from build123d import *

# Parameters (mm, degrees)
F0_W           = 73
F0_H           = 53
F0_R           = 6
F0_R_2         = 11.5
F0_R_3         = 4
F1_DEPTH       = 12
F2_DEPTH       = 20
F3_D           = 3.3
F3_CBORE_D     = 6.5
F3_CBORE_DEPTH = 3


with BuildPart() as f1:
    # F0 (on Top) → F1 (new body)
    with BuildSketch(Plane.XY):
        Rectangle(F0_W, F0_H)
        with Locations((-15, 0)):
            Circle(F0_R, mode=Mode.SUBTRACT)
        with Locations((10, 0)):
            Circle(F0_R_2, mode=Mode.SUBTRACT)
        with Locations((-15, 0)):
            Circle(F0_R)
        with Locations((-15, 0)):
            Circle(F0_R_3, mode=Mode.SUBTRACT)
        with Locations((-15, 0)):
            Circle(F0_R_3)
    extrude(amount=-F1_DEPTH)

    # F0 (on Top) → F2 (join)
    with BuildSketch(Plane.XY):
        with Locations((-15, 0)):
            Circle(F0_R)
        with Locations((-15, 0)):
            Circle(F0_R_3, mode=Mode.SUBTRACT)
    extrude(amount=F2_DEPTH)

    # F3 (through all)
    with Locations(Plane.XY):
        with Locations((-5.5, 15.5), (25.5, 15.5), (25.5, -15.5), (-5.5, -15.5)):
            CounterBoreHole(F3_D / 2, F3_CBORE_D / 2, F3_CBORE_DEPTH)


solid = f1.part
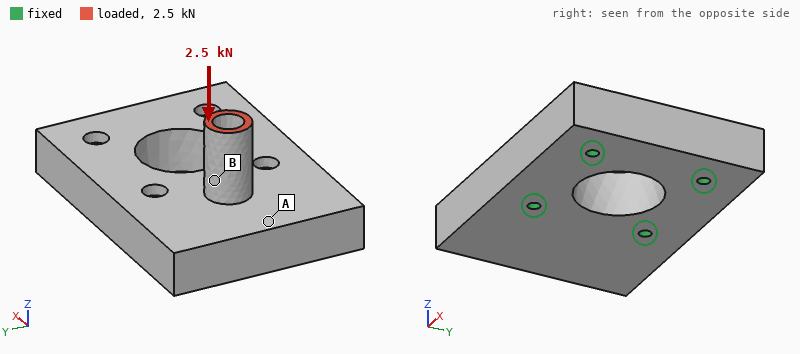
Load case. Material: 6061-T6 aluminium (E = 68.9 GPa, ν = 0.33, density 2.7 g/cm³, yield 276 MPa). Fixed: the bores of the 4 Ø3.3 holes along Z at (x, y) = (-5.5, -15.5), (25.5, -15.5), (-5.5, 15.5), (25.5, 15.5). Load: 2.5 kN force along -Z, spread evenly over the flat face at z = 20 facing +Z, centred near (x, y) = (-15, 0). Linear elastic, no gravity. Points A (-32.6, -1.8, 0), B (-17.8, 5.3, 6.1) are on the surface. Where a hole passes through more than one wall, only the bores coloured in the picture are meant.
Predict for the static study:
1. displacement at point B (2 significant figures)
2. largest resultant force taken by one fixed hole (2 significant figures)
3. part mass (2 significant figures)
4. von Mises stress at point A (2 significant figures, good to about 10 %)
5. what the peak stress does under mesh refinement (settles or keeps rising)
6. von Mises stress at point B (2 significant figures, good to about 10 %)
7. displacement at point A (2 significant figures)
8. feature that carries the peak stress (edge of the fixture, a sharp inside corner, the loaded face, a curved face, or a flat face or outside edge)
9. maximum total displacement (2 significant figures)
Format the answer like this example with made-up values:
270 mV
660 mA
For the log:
20 µm
1.4 kN
110 g
7.3 MPa
keeps rising
39 MPa
23 µm
edge of the fixture
34 µm
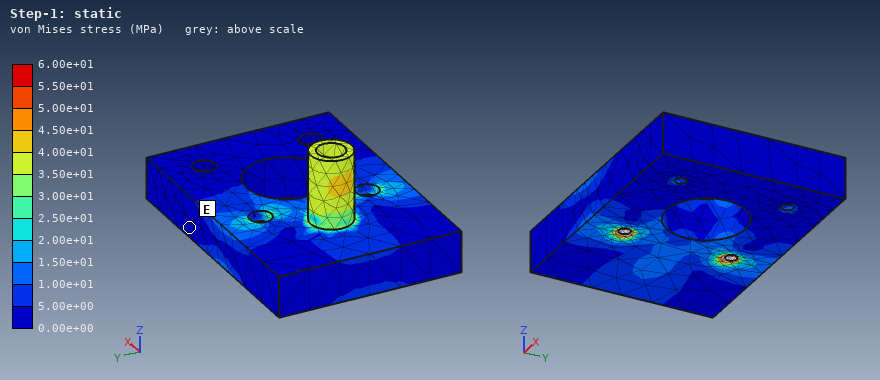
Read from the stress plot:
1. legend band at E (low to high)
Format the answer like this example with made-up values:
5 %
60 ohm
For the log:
0.00e+00 to 5.00e+00 MPa
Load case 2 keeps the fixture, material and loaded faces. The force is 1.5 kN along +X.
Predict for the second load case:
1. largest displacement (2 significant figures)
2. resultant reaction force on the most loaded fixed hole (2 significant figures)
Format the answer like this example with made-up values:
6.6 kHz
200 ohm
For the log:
0.18 mm
670 N
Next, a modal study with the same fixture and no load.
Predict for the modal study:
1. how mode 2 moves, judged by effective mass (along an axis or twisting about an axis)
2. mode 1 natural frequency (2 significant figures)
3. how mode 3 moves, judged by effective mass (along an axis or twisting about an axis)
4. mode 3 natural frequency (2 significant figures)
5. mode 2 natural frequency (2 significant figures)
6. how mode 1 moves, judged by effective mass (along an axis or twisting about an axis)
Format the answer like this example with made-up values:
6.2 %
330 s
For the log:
twisting about X
6300 Hz
along Y
16 kHz
12 kHz
along Z
